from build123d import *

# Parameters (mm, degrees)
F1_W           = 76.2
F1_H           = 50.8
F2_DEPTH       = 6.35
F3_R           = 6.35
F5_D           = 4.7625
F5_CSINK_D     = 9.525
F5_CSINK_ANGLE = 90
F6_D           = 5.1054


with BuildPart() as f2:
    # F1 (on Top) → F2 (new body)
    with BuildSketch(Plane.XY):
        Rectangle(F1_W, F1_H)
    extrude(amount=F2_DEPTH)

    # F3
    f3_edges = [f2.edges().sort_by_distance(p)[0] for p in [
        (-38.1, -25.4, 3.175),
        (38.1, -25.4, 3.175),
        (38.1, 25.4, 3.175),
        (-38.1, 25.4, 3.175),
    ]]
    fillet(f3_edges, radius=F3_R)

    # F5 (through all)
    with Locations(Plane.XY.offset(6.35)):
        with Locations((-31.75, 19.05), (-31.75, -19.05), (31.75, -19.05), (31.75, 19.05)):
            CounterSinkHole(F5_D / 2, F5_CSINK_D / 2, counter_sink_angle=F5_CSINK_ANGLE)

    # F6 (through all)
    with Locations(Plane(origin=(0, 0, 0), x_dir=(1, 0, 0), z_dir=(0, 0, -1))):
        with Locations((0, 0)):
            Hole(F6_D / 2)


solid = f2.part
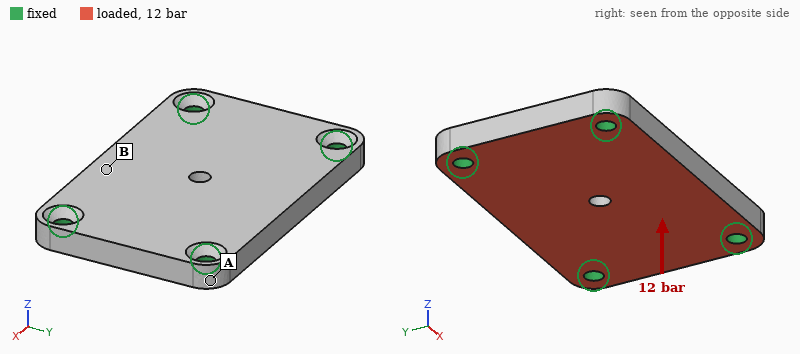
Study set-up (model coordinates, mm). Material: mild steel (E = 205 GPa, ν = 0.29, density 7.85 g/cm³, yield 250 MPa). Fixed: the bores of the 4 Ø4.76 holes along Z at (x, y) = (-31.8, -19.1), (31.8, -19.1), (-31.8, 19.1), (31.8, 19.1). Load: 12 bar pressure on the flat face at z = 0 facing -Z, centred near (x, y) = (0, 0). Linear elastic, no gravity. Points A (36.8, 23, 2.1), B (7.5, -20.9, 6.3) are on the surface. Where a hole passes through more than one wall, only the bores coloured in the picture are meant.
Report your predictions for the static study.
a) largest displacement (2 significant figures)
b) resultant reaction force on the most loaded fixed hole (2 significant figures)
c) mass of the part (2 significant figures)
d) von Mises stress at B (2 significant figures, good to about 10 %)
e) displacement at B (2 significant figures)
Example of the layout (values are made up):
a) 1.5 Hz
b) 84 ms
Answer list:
a) 22 µm
b) 1.2 kN
c) 180 g
d) 39 MPa
e) 18 µm
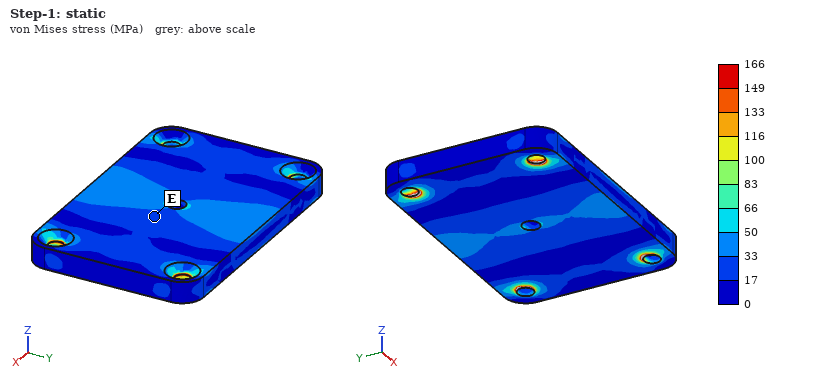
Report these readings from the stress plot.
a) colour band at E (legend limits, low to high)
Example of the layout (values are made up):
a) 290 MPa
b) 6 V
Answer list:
a) 17 to 33 MPa
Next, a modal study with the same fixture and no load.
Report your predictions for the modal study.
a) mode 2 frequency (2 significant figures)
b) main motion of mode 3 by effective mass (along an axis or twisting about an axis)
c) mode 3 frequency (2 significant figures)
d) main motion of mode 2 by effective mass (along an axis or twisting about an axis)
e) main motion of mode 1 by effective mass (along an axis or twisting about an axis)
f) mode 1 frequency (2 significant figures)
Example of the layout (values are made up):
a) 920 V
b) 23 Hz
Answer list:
a) 9200 Hz
b) twisting about Y
c) 15 kHz
d) twisting about X
e) along Z
f) 6100 Hz
